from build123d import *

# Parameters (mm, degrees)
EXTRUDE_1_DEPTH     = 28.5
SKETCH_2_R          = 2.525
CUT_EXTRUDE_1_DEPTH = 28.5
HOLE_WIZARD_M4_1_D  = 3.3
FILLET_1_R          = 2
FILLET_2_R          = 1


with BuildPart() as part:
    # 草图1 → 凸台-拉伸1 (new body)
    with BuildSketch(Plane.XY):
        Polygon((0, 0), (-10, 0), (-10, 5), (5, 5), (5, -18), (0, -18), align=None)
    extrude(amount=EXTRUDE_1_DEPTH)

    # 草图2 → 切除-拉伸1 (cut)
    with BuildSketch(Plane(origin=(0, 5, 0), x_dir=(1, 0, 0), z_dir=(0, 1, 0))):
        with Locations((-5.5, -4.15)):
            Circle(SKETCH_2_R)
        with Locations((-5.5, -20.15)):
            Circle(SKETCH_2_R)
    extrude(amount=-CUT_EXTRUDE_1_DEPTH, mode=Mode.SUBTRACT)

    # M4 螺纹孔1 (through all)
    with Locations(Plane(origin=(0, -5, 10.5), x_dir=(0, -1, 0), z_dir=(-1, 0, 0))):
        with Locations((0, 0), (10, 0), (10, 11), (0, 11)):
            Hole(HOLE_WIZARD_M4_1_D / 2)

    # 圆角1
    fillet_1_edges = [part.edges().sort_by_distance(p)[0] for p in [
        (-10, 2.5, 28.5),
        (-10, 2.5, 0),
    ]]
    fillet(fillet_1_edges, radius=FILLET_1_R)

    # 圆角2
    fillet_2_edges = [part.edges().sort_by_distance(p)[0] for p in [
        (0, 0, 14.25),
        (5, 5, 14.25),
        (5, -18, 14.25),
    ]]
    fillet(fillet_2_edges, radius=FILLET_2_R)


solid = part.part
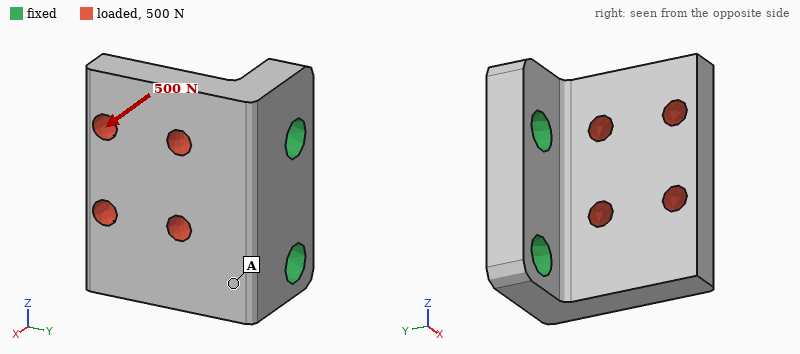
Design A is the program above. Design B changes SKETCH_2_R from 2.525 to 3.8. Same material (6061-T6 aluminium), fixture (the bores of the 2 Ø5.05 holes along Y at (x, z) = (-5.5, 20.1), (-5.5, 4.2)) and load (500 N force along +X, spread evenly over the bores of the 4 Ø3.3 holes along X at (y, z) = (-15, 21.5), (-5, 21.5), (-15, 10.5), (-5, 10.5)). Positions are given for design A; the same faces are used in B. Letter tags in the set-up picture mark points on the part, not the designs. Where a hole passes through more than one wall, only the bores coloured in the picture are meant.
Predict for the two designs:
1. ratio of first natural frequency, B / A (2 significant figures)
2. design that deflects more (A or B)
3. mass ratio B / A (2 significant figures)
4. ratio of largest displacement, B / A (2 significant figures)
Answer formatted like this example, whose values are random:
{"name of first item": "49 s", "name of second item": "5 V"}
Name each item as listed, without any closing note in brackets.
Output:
{"ratio of first natural frequency, B / A": "1.1", "design that deflects more": "A", "mass ratio B / A": "0.94", "ratio of largest displacement, B / A": "0.85"}
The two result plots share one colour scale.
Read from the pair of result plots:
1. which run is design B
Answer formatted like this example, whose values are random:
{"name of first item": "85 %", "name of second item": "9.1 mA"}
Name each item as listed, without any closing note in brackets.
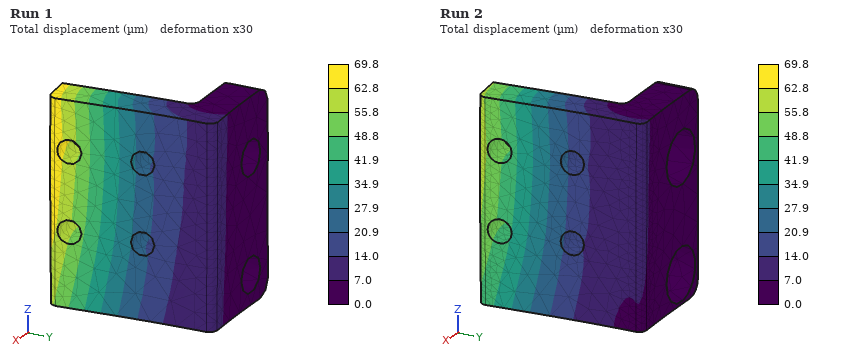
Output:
{"which run is design B": "Run 2"}
